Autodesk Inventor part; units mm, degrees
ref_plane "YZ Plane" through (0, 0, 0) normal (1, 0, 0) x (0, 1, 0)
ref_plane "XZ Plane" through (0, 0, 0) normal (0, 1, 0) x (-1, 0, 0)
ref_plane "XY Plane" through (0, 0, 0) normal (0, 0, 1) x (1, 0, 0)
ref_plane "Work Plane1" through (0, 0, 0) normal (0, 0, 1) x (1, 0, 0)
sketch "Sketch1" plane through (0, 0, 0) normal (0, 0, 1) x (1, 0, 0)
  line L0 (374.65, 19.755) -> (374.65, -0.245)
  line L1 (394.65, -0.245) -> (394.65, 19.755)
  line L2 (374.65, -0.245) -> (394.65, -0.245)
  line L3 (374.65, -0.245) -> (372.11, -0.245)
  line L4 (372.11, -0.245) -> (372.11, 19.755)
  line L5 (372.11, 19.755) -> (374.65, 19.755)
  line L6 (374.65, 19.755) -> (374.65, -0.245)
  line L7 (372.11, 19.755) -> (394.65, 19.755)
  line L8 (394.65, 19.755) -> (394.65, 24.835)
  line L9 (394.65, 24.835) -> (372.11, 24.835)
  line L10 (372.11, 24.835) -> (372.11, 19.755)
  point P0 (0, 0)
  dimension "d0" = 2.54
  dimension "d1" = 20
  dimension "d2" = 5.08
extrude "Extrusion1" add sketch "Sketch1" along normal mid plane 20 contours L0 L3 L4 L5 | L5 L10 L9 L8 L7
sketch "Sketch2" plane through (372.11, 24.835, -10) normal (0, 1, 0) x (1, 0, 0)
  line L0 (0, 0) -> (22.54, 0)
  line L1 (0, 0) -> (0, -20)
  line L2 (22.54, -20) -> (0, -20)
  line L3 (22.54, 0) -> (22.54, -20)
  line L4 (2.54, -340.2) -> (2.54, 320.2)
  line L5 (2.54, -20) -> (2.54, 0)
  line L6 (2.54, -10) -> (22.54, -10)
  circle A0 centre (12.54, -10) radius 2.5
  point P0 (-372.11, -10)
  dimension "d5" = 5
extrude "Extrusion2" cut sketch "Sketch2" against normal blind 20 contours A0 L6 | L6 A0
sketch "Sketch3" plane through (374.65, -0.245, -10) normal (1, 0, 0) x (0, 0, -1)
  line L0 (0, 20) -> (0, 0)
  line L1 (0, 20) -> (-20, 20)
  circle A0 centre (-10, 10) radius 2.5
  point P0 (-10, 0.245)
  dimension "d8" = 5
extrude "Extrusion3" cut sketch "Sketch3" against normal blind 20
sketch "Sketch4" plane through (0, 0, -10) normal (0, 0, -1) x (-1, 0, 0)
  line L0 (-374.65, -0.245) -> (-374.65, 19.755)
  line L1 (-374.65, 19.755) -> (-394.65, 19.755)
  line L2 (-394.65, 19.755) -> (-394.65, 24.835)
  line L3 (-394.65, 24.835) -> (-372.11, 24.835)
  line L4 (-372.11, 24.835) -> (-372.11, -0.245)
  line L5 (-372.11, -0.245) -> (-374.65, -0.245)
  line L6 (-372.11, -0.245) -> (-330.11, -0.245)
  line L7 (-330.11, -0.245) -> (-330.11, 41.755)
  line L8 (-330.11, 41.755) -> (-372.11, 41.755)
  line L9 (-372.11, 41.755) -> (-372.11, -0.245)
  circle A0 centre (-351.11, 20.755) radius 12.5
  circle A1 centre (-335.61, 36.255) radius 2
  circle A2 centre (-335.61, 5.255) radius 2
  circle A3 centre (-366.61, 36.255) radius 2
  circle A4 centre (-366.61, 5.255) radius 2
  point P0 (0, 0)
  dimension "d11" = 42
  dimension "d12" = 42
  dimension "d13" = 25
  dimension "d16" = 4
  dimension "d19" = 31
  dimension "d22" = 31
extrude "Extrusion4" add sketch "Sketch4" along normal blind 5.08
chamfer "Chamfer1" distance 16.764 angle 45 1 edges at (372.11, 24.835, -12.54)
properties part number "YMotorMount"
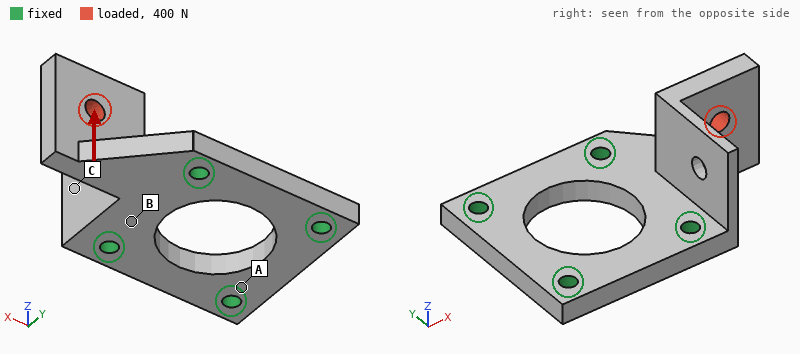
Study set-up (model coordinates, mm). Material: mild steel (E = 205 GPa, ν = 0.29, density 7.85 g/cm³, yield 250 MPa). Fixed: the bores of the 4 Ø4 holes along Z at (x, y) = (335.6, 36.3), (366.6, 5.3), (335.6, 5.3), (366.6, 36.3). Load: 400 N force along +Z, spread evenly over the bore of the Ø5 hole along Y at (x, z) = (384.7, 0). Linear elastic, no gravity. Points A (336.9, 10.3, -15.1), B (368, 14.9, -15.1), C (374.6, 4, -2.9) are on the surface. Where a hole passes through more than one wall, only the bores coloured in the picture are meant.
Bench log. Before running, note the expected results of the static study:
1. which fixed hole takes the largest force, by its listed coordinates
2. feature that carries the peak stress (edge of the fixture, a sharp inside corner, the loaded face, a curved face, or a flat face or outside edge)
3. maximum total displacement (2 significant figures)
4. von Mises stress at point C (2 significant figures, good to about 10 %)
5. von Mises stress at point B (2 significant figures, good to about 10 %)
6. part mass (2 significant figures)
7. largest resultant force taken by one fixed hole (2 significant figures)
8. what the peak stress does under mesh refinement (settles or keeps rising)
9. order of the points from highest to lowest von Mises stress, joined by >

(366.6, 36.3)
edge of the fixture
43 µm
18 MPa
29 MPa
86 g
260 N
keeps rising
B > C > A
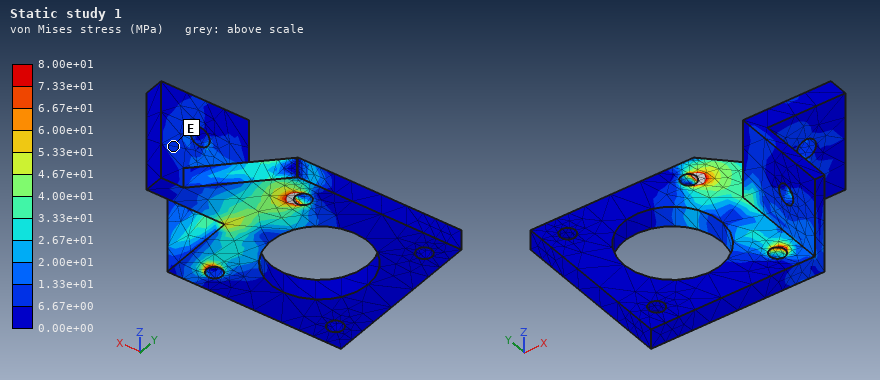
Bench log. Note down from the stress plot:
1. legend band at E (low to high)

6.67e+00 to 1.33e+01 MPa
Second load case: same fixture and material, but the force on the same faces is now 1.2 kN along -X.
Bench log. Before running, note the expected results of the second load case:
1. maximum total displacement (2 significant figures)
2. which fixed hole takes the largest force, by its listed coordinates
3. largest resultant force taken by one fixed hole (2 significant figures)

0.12 mm
(366.6, 36.3)
700 N
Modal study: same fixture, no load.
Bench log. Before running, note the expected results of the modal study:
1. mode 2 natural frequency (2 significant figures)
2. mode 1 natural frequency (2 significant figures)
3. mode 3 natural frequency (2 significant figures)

7400 Hz
3500 Hz
8700 Hz
